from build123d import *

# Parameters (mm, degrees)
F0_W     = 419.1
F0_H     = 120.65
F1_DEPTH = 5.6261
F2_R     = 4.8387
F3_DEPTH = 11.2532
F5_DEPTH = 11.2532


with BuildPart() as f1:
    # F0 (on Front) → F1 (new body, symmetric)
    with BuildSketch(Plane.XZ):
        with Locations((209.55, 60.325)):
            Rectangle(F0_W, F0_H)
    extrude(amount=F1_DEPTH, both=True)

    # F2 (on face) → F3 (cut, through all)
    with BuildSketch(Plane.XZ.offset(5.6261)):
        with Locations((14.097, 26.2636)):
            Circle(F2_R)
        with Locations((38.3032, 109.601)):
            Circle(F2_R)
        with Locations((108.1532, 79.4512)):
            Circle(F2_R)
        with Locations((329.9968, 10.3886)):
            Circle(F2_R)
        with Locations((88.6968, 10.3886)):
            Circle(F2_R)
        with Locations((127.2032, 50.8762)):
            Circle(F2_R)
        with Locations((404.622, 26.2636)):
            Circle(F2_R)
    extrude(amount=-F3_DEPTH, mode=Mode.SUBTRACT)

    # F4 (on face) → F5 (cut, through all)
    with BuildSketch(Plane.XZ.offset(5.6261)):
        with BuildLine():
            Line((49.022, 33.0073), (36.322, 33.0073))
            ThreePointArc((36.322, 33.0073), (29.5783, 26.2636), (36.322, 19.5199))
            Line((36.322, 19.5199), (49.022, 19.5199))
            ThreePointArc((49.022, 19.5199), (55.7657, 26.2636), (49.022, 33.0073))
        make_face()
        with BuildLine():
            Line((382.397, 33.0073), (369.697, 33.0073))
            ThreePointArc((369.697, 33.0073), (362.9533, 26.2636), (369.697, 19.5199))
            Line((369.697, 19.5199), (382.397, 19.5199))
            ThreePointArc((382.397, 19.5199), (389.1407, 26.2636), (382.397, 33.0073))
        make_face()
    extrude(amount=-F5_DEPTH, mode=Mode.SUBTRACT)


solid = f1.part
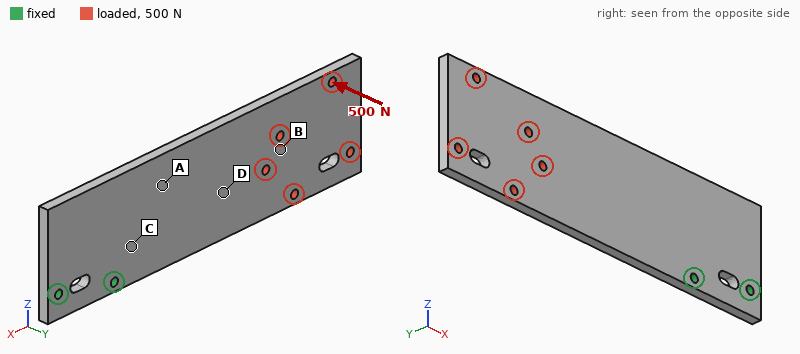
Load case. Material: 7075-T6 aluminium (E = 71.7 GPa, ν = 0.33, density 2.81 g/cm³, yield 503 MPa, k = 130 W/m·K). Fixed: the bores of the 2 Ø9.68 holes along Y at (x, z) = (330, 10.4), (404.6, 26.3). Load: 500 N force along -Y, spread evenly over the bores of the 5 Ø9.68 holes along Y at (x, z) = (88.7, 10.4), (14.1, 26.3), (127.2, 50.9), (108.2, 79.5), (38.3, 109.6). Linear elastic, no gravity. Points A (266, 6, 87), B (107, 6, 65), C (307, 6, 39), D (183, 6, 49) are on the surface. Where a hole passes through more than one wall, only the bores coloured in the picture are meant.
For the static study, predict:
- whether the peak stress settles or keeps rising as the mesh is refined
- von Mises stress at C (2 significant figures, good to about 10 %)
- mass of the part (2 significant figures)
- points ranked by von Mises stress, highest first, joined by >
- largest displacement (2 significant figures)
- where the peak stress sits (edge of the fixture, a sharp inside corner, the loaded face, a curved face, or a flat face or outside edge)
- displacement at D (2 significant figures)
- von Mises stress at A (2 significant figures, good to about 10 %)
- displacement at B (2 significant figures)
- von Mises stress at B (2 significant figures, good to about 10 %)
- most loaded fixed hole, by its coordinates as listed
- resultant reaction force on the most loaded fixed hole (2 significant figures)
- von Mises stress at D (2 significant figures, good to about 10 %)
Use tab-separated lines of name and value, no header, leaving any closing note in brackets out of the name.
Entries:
whether the peak stress settles or keeps rising as the mesh is refined	keeps rising
von Mises stress at C	46 MPa
mass of the part	1.6 kg
points ranked by von Mises stress, highest first, joined by >	C > A > D > B
largest displacement	4.7 mm
where the peak stress sits	edge of the fixture
displacement at D	1.4 mm
von Mises stress at A	35 MPa
displacement at B	2.7 mm
von Mises stress at B	8.0 MPa
most loaded fixed hole, by its coordinates as listed	(330, 10.4)
resultant reaction force on the most loaded fixed hole	1.5 kN
von Mises stress at D	21 MPa
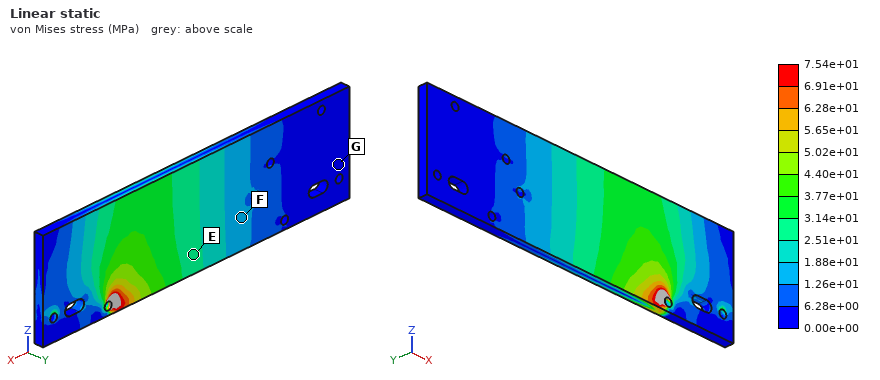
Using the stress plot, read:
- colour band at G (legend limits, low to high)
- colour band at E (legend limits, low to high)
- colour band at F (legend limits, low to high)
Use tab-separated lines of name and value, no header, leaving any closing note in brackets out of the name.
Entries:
colour band at G	0.00e+00 to 6.28e+00 MPa
colour band at E	2.51e+01 to 3.14e+01 MPa
colour band at F	1.26e+01 to 1.88e+01 MPa
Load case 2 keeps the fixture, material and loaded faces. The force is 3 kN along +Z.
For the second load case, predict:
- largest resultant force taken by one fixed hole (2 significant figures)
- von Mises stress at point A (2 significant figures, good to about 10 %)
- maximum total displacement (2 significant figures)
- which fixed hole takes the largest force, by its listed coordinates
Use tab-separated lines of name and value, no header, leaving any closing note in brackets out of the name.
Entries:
largest resultant force taken by one fixed hole	12 kN
von Mises stress at point A	10 MPa
maximum total displacement	0.44 mm
which fixed hole takes the largest force, by its listed coordinates	(330, 10.4)
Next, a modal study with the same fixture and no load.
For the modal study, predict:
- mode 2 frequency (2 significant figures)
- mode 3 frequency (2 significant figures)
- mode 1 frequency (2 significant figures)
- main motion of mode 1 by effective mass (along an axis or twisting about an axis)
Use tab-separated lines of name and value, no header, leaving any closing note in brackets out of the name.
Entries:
mode 2 frequency	350 Hz
mode 3 frequency	490 Hz
mode 1 frequency	77 Hz
main motion of mode 1 by effective mass	along Y
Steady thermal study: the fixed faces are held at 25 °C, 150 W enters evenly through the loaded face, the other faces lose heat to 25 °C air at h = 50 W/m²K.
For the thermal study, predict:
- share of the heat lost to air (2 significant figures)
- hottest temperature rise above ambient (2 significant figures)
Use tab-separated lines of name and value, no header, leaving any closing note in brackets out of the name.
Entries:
share of the heat lost to air	90 %
hottest temperature rise above ambient	61 K
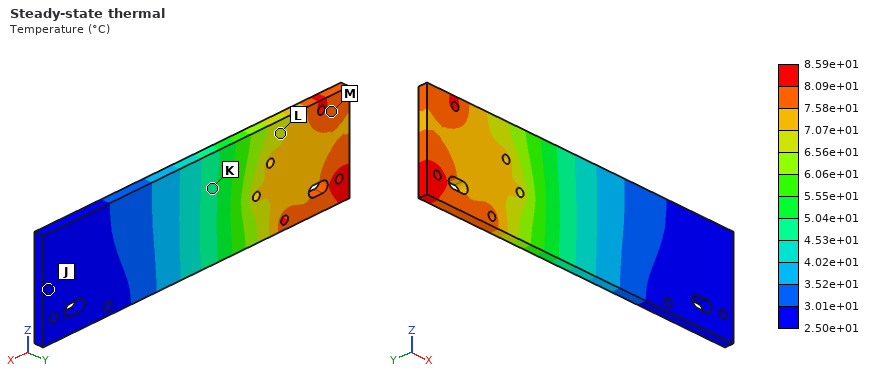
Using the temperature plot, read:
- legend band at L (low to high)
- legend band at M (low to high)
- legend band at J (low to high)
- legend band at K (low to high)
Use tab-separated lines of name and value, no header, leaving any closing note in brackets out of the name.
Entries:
legend band at L	6.56e+01 to 7.07e+01 °C
legend band at M	7.58e+01 to 8.09e+01 °C
legend band at J	2.50e+01 to 3.01e+01 °C
legend band at K	4.53e+01 to 5.04e+01 °C
